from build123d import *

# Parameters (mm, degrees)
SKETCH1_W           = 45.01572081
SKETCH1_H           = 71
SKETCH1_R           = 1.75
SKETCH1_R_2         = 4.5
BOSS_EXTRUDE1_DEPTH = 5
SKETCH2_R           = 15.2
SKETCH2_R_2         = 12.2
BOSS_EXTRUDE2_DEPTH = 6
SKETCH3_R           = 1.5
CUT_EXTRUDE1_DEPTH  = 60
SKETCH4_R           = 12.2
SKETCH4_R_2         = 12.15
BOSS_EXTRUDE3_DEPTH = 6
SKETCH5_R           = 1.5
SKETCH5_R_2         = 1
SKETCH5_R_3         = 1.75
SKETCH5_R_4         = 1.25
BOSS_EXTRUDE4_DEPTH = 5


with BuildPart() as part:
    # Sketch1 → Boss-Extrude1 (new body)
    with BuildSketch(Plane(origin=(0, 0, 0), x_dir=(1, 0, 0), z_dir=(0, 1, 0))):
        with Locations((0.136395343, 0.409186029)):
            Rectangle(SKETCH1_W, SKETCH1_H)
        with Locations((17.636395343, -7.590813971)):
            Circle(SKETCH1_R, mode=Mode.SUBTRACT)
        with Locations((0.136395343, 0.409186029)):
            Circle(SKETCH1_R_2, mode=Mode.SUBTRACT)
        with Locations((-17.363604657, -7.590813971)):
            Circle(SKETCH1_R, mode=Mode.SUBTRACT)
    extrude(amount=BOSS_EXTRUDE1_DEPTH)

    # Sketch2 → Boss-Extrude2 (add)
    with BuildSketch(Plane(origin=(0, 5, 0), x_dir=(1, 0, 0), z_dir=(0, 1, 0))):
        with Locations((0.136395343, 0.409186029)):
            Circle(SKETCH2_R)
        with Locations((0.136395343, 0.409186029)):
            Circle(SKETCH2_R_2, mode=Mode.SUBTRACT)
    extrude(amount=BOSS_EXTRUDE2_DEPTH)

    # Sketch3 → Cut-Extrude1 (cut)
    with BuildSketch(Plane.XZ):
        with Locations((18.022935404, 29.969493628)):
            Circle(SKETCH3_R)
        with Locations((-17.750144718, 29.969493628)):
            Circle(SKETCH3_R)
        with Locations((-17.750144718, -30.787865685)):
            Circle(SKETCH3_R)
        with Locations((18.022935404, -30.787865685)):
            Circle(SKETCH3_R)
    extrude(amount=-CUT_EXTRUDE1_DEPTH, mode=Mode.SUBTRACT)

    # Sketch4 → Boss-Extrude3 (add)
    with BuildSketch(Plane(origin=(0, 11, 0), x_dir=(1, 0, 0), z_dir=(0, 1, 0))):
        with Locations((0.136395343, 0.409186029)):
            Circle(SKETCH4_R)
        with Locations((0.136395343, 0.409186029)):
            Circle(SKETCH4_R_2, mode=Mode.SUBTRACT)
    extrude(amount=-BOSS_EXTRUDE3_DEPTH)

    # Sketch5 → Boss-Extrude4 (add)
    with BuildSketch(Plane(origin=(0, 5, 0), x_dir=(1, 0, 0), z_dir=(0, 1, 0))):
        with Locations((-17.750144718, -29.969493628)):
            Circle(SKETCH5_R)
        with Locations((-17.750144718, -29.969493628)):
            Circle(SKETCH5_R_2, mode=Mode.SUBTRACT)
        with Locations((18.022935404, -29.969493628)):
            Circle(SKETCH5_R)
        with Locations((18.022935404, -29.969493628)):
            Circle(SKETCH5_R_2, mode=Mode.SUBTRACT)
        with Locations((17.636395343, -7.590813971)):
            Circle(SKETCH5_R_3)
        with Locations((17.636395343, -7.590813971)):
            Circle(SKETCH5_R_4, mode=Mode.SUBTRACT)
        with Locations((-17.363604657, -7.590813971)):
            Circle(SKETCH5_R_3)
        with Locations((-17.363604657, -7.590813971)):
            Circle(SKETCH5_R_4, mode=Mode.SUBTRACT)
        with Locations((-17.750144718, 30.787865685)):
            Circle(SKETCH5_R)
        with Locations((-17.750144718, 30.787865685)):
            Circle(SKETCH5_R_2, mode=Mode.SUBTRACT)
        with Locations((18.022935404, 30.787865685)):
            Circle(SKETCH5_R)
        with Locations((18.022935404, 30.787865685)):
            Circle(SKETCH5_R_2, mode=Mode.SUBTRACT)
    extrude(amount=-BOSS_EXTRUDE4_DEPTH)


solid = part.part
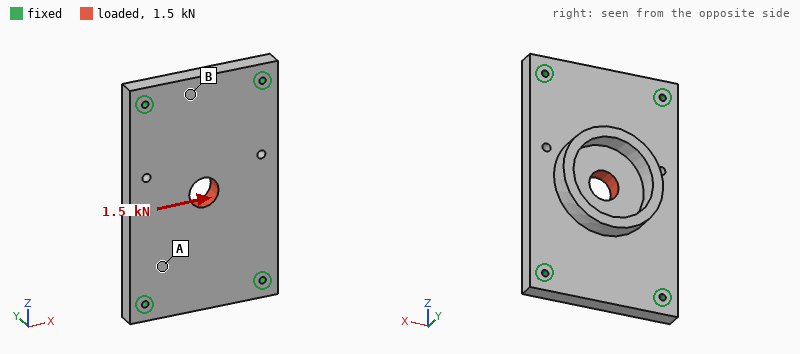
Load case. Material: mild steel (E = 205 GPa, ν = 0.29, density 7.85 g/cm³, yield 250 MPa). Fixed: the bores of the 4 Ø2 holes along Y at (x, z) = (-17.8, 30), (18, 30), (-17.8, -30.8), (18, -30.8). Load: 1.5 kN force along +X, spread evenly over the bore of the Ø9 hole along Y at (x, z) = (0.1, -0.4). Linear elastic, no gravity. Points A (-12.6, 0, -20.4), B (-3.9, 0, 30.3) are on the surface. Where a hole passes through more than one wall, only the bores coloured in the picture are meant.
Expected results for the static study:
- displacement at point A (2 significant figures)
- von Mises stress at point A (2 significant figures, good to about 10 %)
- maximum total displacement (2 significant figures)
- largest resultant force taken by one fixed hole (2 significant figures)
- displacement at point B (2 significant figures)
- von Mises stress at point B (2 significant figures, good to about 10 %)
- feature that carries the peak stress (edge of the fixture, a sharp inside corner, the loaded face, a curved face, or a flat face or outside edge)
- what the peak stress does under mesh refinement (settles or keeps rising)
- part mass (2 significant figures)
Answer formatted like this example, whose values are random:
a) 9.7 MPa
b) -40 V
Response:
a) 0.79 µm
b) 7.2 MPa
c) 2.0 µm
d) 480 N
e) 0.32 µm
f) 2.9 MPa
g) edge of the fixture
h) keeps rising
i) 130 g
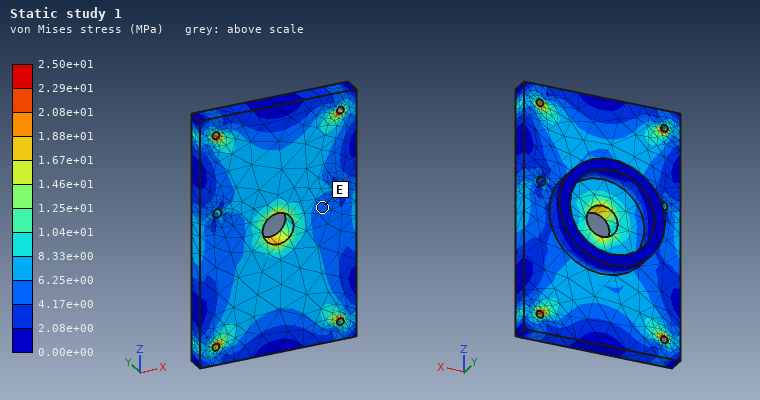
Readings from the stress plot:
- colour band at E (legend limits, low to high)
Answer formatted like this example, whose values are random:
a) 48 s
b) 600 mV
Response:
a) 4.17e+00 to 6.25e+00 MPa
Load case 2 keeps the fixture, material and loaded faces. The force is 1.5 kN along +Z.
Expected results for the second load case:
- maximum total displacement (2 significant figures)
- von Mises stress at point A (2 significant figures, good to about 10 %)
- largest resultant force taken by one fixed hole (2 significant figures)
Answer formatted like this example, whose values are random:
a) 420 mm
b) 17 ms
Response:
a) 1.1 µm
b) 5.4 MPa
c) 390 N
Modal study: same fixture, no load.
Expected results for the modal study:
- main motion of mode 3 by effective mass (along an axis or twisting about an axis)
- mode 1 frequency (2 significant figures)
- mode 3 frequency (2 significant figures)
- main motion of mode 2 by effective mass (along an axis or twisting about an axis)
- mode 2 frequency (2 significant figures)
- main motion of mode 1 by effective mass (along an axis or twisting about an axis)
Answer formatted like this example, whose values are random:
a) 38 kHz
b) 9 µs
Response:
a) twisting about X
b) 5500 Hz
c) 13 kHz
d) twisting about Z
e) 8300 Hz
f) along Y
